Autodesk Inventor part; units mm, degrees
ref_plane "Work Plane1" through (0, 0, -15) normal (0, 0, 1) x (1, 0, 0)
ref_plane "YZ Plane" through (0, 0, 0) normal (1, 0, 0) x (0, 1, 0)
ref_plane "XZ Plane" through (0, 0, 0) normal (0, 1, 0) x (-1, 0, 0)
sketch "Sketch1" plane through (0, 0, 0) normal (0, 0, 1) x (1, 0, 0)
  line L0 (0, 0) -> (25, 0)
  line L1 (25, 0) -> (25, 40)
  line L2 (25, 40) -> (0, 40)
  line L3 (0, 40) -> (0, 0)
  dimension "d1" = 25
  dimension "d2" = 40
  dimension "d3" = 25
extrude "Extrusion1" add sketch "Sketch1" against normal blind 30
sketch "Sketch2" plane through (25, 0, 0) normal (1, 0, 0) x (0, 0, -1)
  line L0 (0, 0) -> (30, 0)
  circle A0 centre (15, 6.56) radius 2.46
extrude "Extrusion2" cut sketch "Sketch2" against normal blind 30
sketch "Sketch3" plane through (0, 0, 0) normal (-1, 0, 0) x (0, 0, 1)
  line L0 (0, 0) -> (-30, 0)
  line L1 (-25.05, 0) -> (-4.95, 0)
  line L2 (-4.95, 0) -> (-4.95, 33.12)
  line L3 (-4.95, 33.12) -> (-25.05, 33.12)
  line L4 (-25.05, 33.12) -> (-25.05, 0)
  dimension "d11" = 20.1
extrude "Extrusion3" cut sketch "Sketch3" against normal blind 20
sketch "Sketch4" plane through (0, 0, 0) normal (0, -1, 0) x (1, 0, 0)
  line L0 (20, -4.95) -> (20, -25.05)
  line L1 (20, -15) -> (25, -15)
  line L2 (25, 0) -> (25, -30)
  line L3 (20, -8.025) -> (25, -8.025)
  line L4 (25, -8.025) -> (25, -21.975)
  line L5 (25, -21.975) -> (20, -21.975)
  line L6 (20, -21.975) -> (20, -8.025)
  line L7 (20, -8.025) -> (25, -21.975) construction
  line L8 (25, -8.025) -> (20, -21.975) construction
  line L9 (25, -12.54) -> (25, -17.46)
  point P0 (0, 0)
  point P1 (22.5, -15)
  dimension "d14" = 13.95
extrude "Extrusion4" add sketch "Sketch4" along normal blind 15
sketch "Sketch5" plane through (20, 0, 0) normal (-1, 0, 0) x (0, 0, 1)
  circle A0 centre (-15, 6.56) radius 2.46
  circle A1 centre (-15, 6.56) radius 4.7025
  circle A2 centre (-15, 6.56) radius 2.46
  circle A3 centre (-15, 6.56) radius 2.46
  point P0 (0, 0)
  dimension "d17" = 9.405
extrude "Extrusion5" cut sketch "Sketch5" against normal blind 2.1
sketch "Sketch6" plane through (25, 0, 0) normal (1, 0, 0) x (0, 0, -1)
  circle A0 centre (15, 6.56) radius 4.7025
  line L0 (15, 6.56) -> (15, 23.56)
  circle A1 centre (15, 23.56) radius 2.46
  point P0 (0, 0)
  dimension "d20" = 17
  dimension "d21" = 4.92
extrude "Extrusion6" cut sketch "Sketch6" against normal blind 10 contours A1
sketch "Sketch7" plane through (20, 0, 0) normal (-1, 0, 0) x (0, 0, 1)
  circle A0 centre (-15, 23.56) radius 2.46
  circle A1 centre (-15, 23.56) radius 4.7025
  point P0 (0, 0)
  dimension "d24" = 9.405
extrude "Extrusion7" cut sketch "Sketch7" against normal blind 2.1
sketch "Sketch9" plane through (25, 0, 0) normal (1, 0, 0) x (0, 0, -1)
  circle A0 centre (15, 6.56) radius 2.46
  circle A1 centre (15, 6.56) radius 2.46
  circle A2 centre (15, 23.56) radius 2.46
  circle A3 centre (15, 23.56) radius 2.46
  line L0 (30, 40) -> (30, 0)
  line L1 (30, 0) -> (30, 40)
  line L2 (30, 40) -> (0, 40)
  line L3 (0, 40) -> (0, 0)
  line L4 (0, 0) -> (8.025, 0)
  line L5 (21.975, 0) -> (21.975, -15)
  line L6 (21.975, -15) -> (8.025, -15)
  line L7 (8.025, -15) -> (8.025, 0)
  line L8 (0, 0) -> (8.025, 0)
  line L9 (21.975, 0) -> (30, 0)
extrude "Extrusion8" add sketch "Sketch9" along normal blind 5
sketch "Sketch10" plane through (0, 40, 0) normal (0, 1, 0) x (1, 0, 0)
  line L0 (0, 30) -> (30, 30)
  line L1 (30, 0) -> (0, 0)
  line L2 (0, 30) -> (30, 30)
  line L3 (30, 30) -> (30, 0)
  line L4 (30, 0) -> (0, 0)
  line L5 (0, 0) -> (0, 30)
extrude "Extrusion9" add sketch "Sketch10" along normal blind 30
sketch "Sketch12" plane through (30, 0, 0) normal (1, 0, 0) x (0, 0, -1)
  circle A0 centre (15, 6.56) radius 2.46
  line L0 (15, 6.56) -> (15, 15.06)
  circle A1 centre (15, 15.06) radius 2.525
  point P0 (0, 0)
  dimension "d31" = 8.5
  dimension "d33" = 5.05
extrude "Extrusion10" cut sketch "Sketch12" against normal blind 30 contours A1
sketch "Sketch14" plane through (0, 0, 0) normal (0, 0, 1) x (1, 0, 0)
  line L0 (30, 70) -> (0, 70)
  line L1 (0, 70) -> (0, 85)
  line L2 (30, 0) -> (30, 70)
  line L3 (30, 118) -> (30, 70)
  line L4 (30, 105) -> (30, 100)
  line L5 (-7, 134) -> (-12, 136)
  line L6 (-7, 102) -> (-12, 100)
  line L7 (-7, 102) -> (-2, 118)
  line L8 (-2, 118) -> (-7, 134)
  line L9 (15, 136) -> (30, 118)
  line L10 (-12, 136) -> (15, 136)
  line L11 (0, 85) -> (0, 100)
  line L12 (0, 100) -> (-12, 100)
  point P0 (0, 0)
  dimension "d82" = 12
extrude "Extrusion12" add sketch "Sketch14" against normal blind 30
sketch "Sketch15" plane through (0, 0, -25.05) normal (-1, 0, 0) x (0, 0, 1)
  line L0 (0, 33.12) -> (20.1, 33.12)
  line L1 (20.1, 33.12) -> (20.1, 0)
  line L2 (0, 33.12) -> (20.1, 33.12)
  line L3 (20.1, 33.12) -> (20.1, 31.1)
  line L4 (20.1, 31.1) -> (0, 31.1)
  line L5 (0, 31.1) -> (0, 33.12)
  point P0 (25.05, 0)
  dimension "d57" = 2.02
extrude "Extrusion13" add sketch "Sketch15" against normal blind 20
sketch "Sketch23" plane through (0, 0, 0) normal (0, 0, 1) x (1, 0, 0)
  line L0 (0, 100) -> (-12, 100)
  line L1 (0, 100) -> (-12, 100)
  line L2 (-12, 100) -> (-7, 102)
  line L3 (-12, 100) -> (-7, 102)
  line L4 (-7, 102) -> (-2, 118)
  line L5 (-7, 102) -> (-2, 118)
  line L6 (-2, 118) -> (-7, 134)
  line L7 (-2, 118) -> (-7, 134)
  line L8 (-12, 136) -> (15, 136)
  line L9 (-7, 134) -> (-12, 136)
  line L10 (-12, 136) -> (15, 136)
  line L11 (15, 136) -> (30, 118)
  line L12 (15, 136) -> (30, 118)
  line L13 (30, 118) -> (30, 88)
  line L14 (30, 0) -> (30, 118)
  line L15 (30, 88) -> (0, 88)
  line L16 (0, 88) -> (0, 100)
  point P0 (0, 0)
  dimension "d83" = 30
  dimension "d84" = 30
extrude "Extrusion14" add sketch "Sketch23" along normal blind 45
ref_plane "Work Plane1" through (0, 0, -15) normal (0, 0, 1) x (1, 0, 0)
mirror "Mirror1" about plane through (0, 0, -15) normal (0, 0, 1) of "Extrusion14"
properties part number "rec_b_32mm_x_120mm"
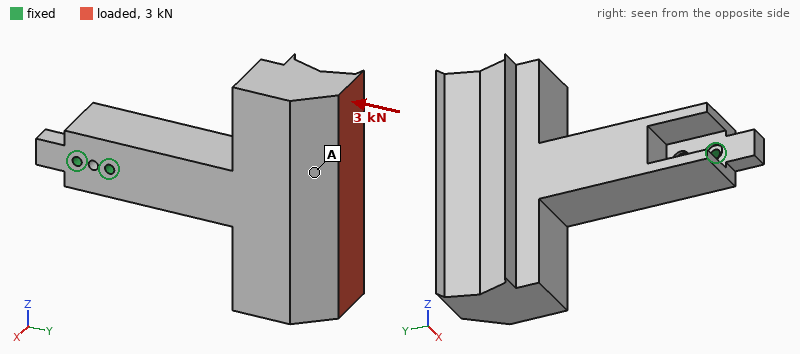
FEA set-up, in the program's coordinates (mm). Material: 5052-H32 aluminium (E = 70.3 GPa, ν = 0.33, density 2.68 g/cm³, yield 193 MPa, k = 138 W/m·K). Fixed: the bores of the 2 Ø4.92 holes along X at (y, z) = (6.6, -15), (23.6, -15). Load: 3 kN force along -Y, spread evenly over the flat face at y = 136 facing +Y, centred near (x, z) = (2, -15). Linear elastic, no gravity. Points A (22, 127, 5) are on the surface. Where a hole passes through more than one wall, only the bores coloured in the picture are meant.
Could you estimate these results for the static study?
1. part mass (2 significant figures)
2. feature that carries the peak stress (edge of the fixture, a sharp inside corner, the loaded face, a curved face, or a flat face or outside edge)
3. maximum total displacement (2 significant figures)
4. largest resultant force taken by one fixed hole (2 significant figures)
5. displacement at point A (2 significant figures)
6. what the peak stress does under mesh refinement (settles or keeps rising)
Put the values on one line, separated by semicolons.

660 g; edge of the fixture; 0.23 mm; 3.4 kN; 0.20 mm; keeps rising
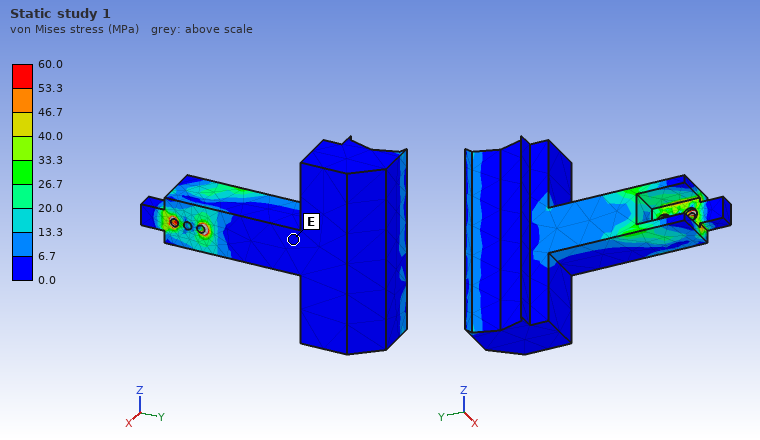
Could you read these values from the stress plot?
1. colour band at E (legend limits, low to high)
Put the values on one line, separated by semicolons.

0.0 to 6.7 MPa
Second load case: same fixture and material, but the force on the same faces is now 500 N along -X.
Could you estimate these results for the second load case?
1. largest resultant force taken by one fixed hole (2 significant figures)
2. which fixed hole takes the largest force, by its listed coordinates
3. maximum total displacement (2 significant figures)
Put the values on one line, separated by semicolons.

2.8 kN; (23.6, -15); 0.19 mm
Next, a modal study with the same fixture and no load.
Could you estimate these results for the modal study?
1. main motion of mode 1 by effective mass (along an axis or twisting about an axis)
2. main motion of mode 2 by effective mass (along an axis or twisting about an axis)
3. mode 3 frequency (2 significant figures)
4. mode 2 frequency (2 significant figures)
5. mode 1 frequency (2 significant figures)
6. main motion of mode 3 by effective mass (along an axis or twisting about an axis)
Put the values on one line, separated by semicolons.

along X; along Z; 770 Hz; 520 Hz; 480 Hz; twisting about Y
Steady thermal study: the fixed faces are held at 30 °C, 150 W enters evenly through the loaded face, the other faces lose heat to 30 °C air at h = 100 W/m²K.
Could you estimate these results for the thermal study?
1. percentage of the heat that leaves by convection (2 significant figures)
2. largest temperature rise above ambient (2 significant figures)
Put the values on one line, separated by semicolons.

72 %; 59 K
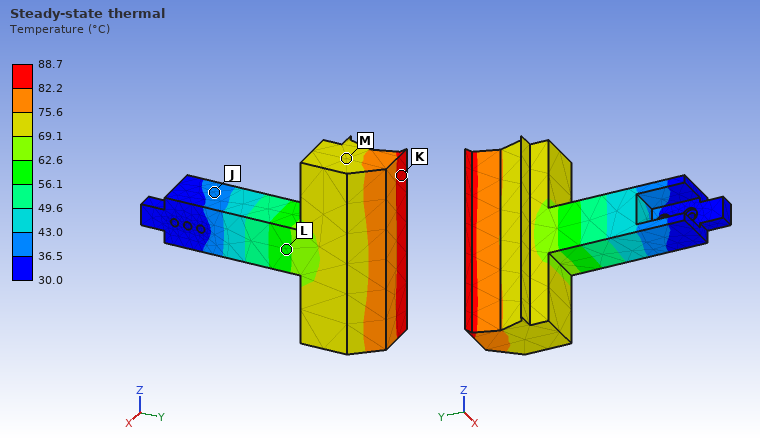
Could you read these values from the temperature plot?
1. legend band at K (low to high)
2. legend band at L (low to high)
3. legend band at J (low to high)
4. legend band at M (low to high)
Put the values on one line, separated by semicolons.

82.2 to 88.7 °C; 56.1 to 62.6 °C; 36.5 to 43.0 °C; 69.1 to 75.6 °C
